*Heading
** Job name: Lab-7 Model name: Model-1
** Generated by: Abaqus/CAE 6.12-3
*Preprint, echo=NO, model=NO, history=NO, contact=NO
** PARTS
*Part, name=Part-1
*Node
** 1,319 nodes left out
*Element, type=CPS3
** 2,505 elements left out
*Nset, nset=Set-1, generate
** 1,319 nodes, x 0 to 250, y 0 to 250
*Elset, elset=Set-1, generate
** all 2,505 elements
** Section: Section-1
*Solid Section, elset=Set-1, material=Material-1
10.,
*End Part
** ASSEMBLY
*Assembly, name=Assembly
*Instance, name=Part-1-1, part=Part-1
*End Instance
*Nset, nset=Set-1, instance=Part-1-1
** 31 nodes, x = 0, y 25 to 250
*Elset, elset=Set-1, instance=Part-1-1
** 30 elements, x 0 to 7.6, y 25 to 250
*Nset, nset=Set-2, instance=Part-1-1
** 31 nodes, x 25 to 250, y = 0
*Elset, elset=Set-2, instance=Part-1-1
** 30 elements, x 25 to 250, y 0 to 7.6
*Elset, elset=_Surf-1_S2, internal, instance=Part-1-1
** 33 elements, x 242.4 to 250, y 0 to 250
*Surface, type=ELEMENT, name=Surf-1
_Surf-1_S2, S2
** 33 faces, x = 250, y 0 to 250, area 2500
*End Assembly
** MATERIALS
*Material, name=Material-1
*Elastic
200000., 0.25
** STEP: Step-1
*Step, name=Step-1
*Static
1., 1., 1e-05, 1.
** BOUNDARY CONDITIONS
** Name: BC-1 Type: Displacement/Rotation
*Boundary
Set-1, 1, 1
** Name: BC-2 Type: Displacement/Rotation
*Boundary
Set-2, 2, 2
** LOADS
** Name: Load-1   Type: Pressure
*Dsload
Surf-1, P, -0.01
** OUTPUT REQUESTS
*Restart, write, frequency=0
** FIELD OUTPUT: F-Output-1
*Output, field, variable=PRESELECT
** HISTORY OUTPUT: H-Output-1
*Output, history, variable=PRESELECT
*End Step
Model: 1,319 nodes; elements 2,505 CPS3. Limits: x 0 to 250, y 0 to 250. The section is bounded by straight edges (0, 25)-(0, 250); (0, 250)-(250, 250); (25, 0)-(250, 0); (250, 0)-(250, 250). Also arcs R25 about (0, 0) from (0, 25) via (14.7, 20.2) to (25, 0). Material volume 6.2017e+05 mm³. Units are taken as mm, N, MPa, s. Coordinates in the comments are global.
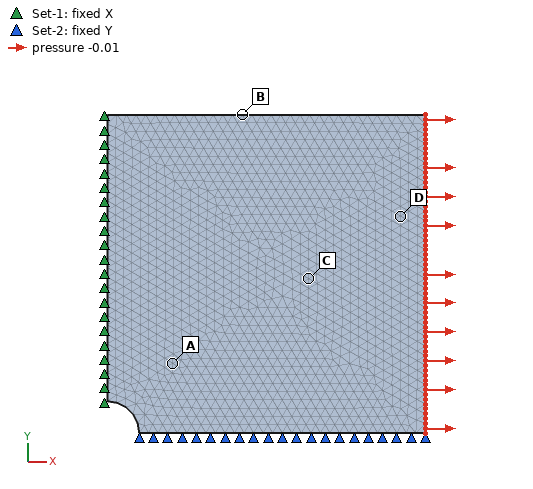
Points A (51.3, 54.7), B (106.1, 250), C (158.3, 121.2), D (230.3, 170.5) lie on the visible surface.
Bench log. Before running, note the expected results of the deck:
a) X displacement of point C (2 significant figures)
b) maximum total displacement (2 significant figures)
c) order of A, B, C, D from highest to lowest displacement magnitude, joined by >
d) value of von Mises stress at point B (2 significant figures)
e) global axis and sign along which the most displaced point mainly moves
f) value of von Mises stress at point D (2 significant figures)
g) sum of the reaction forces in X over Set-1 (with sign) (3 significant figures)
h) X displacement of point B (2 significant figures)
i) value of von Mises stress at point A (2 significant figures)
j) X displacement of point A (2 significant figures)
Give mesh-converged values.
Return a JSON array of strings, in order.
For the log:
["8.2e-06 mm", "1.3e-05 mm", "D > C > B > A", "0.0099 MPa", "+X", "0.010 MPa", "-25.0 N", "5.2e-06 mm", "0.012 MPa", "3.0e-06 mm"]
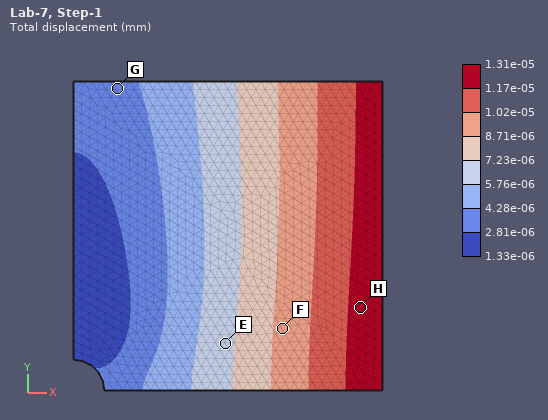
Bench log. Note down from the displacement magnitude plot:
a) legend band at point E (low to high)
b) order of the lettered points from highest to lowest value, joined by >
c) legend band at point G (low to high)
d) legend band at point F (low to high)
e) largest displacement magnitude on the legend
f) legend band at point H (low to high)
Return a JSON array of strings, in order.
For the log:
["5.76e-06 to 7.23e-06 mm", "H > F > E > G", "2.81e-06 to 4.28e-06 mm", "8.71e-06 to 1.02e-05 mm", "1.31e-05 mm", "1.17e-05 to 1.31e-05 mm"]
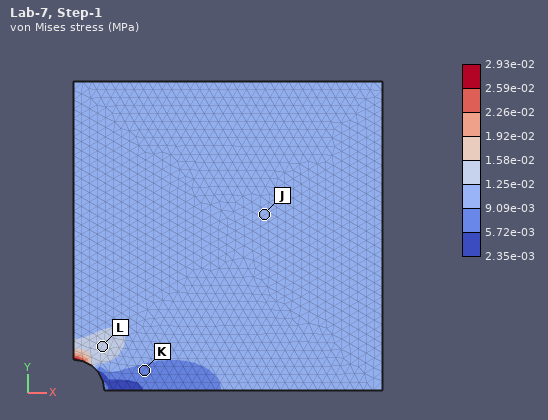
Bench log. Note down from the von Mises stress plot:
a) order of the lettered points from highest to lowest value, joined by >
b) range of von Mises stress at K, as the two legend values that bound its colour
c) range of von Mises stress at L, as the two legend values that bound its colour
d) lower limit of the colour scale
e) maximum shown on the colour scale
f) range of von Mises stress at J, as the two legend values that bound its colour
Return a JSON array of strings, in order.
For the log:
["L > J > K", "5.72e-03 to 9.09e-03 MPa", "1.25e-02 to 1.58e-02 MPa", "2.35e-03 MPa", "2.93e-02 MPa", "9.09e-03 to 1.25e-02 MPa"]
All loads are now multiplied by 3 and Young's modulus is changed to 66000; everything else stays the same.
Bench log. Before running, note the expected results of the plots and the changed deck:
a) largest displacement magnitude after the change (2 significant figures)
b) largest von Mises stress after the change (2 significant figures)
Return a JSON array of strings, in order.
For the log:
["1.2e-04 mm", "0.088 MPa"]
